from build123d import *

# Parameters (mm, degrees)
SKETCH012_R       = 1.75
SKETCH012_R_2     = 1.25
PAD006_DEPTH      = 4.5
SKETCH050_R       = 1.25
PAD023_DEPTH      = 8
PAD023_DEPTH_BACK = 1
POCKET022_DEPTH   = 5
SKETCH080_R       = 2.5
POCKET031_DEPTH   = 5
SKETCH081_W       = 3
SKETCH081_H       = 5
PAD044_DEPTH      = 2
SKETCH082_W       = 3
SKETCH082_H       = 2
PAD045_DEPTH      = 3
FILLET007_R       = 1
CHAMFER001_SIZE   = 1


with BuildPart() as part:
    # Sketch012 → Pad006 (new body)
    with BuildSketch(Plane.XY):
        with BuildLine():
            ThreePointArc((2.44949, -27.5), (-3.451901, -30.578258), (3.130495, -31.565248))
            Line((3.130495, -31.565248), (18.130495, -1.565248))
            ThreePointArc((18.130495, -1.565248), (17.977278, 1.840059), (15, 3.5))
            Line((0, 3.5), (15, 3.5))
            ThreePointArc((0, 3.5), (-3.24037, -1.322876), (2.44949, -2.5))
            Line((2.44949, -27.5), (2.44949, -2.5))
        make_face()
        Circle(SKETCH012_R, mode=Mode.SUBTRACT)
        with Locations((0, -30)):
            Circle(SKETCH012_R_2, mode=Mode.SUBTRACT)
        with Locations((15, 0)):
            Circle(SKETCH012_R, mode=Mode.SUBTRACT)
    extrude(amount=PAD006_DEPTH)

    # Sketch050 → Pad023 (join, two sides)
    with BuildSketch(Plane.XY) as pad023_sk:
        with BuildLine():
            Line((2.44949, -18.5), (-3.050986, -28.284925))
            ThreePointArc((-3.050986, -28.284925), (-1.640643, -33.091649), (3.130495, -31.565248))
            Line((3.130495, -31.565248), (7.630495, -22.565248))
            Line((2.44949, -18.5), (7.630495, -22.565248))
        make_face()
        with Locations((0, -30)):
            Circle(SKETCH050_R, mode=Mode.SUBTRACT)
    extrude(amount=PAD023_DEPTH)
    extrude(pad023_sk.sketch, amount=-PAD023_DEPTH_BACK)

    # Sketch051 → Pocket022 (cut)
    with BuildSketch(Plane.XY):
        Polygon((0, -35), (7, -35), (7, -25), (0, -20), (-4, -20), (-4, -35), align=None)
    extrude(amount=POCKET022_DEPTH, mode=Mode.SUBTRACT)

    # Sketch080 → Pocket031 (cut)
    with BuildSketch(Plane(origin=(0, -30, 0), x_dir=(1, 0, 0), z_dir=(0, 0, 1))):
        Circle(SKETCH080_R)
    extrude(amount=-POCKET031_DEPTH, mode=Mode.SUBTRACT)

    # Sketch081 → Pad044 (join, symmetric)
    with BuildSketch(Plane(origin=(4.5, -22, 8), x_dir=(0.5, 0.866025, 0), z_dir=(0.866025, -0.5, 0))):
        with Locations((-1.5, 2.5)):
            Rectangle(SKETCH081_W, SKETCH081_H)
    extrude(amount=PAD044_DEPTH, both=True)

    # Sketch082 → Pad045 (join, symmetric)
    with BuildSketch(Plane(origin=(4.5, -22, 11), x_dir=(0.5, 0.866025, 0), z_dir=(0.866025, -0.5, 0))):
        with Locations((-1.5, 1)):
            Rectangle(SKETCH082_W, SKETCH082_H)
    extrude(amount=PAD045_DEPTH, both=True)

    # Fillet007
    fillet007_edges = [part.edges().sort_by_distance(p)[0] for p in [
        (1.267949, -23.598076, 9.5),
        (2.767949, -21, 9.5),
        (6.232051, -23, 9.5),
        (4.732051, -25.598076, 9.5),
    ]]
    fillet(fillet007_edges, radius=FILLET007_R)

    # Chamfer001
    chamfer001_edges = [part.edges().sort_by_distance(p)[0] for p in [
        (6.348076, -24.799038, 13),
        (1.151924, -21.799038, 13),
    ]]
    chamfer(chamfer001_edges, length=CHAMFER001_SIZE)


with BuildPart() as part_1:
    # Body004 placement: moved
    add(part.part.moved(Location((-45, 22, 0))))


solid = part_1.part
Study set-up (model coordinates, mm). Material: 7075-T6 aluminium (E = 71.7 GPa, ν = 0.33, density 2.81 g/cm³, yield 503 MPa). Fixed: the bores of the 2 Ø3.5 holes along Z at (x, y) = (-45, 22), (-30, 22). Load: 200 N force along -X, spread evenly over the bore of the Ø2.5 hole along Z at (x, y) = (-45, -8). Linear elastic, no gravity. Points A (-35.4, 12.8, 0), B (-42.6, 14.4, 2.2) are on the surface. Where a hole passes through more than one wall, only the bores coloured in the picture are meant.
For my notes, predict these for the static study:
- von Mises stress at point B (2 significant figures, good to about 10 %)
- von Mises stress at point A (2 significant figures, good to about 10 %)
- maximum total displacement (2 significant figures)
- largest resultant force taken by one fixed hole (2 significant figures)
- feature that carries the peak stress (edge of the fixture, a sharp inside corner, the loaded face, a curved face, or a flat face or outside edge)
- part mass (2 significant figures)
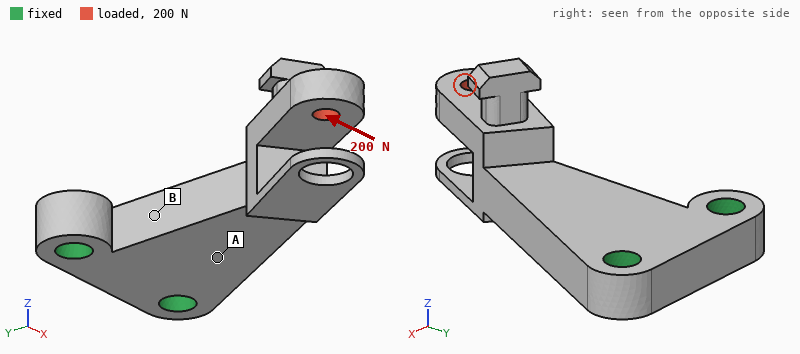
46 MPa
22 MPa
0.14 mm
430 N
a flat face or outside edge
5.2 g
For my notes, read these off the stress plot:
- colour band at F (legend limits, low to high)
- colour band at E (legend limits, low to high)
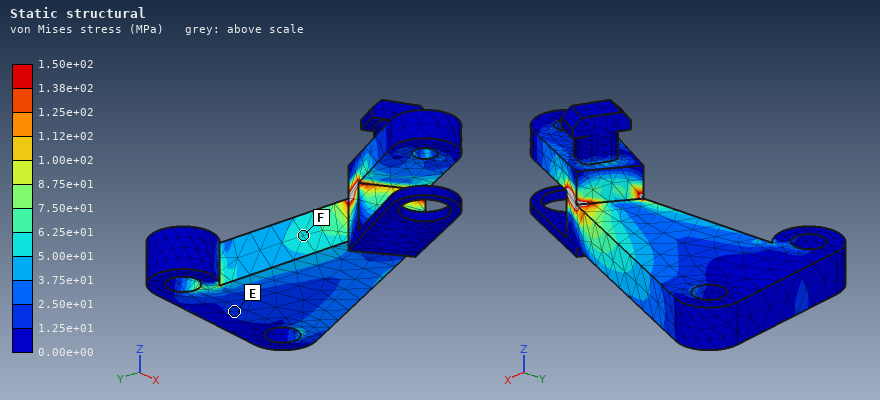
5.00e+01 to 6.25e+01 MPa
1.25e+01 to 2.50e+01 MPa
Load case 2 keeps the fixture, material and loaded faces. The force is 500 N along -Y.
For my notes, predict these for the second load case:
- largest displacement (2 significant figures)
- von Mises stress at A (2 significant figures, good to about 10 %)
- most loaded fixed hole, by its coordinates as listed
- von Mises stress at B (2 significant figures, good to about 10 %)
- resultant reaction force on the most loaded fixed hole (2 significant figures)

0.27 mm
58 MPa
(-45, 22)
50 MPa
530 N
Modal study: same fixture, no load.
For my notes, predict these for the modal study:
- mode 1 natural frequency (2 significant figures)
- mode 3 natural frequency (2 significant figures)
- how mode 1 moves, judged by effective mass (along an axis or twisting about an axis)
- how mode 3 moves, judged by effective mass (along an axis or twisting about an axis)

3700 Hz
8400 Hz
along Z
along X
